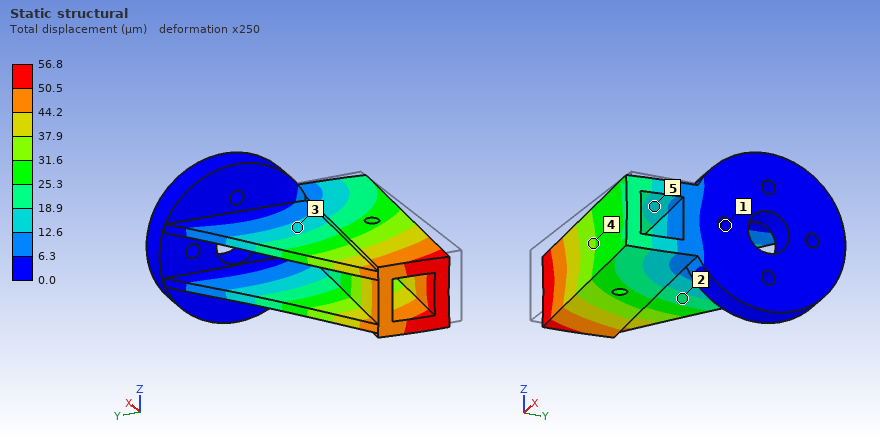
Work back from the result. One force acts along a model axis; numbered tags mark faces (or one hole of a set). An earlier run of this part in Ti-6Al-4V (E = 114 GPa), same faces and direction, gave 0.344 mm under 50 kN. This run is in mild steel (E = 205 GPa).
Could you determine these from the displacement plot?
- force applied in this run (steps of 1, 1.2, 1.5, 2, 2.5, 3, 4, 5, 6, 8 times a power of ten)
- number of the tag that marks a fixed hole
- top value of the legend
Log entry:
15 kN
1
56.8 µm
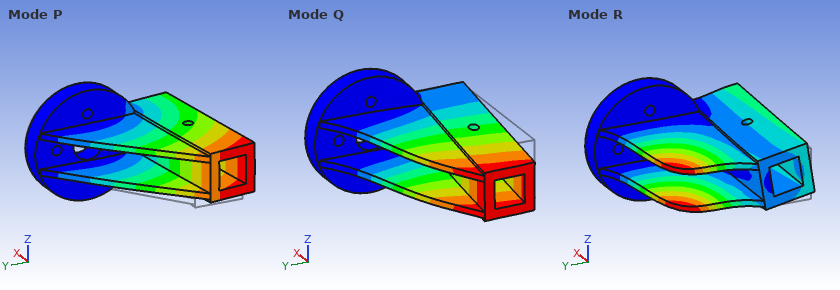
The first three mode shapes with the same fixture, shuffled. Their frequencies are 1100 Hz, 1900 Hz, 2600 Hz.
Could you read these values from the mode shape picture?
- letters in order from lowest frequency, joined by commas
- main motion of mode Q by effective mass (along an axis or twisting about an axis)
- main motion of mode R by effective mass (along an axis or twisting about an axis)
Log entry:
Q, P, R
along Z
twisting about X
